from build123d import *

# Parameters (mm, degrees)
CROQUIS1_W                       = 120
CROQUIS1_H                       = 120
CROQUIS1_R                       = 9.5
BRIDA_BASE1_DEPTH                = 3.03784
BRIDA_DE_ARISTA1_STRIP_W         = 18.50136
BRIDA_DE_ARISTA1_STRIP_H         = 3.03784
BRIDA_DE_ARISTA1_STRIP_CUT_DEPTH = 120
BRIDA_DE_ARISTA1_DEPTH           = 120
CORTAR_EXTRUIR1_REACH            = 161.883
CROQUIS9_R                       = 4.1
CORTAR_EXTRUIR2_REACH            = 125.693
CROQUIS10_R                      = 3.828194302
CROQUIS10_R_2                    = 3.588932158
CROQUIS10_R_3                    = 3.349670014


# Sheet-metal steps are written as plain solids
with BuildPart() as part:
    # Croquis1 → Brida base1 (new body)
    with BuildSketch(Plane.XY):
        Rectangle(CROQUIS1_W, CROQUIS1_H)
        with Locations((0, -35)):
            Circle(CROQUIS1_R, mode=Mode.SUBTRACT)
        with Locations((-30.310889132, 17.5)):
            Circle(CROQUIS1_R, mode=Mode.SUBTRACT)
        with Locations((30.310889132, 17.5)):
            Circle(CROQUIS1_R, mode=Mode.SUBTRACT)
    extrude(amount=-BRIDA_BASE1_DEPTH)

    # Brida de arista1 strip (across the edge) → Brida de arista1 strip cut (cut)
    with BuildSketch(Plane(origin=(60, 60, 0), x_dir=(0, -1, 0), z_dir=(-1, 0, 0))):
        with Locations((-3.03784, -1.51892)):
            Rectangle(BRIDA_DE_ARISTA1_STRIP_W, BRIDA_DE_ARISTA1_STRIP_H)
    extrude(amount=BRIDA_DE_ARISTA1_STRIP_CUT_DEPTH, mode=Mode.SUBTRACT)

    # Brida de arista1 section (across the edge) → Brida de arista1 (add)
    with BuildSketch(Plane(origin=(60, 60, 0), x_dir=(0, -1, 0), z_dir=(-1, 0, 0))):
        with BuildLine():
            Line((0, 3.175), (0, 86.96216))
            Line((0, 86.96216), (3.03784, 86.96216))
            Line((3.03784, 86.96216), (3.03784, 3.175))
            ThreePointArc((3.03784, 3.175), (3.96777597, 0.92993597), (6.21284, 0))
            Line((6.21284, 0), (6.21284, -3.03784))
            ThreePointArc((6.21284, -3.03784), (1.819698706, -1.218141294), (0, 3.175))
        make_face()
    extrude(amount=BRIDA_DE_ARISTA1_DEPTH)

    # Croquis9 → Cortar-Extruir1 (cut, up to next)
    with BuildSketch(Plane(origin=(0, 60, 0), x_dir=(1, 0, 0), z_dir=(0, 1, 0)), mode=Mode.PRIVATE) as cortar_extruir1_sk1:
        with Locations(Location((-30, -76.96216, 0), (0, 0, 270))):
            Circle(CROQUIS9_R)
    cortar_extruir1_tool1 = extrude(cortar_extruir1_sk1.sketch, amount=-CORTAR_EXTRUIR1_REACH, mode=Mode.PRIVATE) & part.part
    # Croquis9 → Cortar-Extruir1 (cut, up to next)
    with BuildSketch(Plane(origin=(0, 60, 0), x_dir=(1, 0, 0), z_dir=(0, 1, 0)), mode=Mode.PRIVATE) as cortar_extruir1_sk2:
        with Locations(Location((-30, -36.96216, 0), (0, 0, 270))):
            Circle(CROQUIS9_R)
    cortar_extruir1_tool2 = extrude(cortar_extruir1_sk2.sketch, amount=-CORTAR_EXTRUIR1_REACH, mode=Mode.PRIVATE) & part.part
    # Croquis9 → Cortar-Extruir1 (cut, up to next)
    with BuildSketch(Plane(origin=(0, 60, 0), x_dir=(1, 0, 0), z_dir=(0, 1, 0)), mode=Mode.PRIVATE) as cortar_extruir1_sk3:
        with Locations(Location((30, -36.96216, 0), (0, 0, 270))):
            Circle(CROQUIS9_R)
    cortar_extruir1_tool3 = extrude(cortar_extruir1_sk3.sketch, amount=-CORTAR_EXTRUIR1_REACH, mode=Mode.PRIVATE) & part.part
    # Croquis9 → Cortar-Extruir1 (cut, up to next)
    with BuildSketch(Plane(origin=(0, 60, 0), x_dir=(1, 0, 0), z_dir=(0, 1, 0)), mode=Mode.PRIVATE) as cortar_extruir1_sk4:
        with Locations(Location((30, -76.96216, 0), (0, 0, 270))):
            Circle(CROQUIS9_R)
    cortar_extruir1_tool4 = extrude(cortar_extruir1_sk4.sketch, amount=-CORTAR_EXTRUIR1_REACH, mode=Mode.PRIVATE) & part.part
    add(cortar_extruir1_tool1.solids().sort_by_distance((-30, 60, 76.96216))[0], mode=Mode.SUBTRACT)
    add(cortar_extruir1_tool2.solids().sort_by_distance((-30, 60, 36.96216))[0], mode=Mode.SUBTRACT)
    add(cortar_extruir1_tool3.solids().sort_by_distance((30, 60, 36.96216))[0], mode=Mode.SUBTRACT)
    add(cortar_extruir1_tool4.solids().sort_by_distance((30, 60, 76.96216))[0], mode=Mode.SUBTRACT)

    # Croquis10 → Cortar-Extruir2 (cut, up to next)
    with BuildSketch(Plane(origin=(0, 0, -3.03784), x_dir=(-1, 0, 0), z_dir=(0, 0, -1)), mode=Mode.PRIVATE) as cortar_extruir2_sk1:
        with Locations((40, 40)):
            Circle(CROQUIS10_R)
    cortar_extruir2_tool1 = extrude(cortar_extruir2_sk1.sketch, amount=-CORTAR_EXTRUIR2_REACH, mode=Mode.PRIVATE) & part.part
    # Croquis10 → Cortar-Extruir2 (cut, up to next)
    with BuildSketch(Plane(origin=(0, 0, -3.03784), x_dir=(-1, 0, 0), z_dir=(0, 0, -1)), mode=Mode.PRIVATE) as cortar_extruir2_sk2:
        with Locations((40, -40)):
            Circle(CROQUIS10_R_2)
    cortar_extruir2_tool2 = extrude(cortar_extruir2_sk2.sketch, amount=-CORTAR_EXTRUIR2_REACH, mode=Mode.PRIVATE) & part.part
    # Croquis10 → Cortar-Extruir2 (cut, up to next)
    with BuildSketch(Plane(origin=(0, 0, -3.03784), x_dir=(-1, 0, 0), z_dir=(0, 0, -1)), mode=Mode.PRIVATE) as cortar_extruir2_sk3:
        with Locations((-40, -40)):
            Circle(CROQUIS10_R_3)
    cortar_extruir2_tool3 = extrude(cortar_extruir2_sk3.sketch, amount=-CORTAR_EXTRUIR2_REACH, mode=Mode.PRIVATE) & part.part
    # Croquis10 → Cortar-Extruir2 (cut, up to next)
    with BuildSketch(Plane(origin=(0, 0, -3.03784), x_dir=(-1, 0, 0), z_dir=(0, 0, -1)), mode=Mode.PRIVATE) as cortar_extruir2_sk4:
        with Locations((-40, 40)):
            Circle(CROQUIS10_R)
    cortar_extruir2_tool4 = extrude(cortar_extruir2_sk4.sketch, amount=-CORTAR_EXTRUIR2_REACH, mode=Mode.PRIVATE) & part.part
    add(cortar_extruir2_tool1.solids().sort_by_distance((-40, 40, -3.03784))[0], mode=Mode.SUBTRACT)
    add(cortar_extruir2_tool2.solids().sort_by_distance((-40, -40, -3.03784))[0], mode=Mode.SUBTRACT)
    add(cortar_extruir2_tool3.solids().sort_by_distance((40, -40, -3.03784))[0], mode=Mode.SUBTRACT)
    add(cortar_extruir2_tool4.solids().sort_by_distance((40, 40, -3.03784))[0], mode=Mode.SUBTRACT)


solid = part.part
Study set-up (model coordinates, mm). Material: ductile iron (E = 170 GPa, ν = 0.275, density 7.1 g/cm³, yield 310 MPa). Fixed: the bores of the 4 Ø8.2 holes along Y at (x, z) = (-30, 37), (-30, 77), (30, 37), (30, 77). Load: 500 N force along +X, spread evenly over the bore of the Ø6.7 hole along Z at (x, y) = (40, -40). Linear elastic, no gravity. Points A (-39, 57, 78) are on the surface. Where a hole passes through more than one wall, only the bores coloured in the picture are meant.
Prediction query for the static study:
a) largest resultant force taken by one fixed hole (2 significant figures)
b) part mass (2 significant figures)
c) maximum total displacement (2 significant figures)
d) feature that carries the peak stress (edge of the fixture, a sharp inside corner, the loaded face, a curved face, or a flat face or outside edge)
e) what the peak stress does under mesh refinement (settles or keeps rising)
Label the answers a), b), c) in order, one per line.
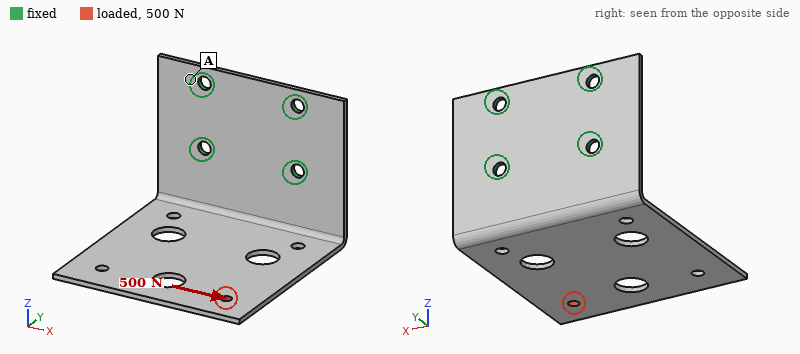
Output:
a) 820 N
b) 500 g
c) 1.1 mm
d) edge of the fixture
e) keeps rising
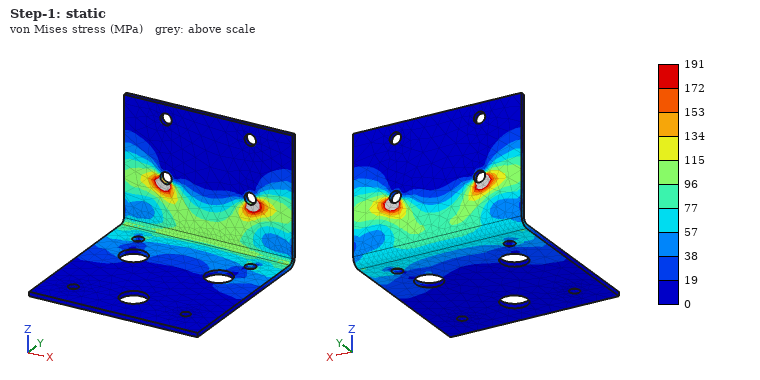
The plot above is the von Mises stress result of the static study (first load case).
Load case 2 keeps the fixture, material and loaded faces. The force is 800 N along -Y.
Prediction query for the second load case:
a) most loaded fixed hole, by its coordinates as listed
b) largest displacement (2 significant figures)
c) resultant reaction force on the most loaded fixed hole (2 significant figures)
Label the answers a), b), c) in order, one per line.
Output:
a) (30, 37)
b) 1.9 mm
c) 980 N
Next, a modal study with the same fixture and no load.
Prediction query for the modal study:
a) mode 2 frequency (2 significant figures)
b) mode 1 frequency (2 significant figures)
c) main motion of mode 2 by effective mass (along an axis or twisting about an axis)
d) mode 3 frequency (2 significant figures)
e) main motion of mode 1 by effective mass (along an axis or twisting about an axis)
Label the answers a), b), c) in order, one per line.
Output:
a) 280 Hz
b) 120 Hz
c) along X
d) 420 Hz
e) along Z
